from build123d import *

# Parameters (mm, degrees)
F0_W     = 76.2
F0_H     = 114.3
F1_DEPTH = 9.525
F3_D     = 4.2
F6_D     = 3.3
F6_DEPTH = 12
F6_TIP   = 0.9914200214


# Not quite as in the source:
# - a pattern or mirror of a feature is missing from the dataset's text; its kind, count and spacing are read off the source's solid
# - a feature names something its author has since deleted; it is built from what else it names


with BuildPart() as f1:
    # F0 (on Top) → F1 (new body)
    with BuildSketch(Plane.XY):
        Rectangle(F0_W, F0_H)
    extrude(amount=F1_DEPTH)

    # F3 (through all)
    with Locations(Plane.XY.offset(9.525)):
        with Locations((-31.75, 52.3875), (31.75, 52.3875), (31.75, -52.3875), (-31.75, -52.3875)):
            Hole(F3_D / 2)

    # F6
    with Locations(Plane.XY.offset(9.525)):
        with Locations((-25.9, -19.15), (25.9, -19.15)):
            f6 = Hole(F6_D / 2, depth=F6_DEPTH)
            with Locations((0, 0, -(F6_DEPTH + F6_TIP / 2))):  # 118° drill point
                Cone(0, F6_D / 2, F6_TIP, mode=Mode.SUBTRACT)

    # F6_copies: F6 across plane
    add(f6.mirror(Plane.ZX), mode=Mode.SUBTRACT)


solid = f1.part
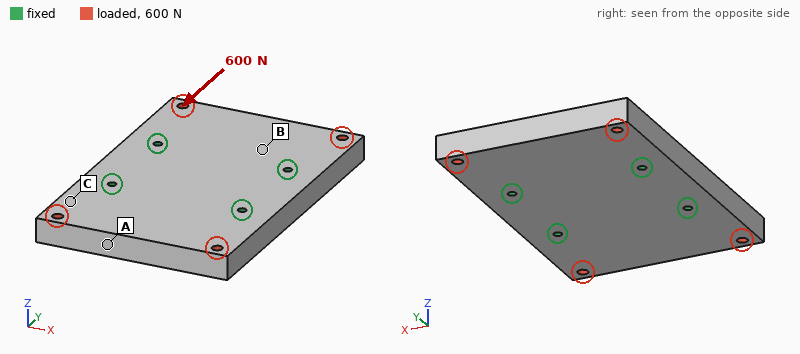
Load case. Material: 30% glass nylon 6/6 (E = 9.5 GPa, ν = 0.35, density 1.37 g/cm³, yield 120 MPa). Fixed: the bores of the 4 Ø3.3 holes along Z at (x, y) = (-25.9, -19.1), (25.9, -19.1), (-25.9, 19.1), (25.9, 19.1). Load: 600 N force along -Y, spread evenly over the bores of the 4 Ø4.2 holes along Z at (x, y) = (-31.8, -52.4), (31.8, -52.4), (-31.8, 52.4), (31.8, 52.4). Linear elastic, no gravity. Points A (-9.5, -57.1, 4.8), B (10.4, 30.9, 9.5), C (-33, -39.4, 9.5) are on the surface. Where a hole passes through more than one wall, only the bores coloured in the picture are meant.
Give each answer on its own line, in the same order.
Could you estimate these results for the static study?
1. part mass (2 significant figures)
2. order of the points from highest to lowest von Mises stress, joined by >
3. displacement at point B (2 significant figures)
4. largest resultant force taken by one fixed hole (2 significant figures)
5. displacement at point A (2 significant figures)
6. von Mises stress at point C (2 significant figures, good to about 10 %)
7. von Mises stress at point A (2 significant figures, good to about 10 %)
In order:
110 g
C > A > B
0.90 µm
150 N
1.2 µm
0.97 MPa
0.55 MPa
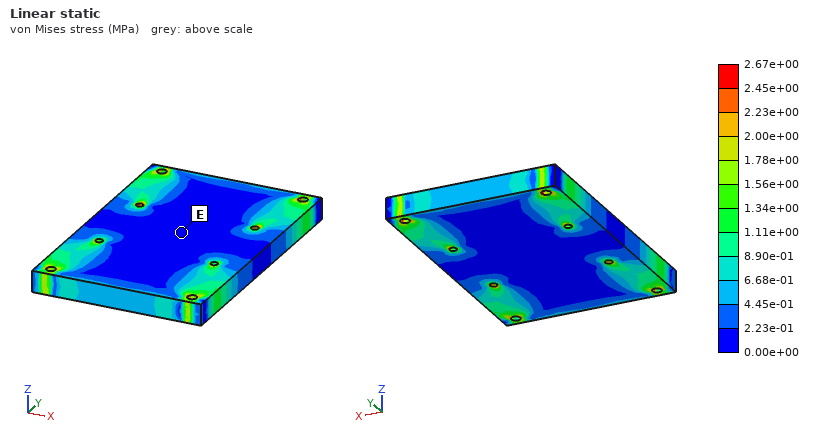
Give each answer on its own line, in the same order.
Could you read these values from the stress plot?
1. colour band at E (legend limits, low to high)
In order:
0.00e+00 to 2.23e-01 MPa
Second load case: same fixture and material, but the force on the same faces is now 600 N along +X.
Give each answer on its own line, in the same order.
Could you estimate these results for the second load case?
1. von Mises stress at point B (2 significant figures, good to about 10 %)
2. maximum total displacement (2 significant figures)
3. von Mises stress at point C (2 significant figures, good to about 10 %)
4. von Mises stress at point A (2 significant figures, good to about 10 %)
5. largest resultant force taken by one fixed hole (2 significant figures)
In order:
1.0 MPa
11 µm
0.44 MPa
0.63 MPa
180 N
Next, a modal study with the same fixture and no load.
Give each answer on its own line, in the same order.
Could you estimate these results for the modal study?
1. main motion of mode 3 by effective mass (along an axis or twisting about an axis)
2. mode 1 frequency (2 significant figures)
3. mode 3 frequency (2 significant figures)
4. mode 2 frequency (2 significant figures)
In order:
twisting about Y
2200 Hz
3700 Hz
2200 Hz
